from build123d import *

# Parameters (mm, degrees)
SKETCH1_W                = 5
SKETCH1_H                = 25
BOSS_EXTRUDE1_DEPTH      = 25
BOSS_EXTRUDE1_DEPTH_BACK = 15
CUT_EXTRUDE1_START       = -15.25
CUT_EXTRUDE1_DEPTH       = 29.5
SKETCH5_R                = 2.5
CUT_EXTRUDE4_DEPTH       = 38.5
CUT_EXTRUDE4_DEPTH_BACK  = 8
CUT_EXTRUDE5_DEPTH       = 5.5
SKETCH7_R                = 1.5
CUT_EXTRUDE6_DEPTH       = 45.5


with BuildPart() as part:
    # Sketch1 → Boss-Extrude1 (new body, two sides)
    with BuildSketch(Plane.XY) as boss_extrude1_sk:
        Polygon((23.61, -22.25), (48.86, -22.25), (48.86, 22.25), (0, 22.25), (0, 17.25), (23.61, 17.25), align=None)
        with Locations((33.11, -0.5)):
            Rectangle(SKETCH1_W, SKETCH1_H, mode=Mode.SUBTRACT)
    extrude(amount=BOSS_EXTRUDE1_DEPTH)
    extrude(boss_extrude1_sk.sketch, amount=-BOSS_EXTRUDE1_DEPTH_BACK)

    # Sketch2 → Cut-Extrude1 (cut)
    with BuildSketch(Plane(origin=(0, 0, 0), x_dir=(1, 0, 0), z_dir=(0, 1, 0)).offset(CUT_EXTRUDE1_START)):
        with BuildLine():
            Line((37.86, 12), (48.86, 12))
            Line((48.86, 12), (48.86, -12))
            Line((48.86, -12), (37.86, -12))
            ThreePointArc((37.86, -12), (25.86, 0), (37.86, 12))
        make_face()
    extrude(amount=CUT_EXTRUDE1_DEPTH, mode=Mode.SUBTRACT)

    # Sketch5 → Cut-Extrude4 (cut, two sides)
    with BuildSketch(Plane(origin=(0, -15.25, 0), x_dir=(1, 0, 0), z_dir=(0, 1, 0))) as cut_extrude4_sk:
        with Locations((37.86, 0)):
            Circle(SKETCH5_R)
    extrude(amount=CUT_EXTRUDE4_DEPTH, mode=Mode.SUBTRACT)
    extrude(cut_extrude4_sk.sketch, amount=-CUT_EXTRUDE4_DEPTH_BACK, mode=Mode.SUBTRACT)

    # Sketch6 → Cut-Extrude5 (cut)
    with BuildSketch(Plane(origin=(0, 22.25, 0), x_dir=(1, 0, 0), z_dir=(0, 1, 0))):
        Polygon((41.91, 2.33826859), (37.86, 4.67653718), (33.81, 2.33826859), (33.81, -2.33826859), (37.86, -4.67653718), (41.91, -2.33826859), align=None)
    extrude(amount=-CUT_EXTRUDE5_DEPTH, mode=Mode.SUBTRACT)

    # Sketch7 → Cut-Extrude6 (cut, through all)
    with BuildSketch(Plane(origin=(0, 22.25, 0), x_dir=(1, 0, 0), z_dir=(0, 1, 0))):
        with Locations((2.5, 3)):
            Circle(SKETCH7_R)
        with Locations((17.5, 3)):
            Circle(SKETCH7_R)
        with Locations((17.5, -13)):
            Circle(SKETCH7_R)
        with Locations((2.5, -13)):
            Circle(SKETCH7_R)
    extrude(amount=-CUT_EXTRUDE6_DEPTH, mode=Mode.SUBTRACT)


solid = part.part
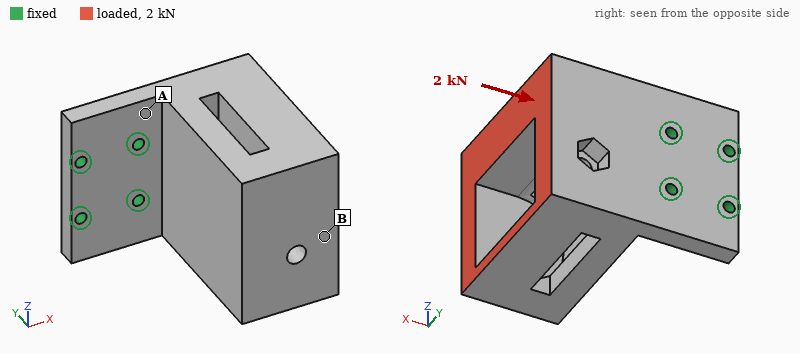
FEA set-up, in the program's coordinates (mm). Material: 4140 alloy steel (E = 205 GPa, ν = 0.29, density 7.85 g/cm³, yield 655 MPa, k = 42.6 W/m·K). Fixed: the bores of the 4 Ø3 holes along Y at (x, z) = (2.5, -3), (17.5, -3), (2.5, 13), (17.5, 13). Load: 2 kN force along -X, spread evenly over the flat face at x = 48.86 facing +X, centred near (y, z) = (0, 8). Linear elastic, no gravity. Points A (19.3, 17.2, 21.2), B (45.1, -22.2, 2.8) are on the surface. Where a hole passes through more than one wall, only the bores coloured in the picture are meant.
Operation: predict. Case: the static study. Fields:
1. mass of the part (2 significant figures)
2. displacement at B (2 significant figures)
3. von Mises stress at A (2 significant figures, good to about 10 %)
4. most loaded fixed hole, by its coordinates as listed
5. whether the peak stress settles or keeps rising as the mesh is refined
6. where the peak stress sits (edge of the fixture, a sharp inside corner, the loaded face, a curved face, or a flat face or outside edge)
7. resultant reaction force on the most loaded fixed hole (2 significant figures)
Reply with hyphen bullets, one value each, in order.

- 250 g
- 0.22 mm
- 170 MPa
- (17.5, 13)
- keeps rising
- edge of the fixture
- 1.2 kN
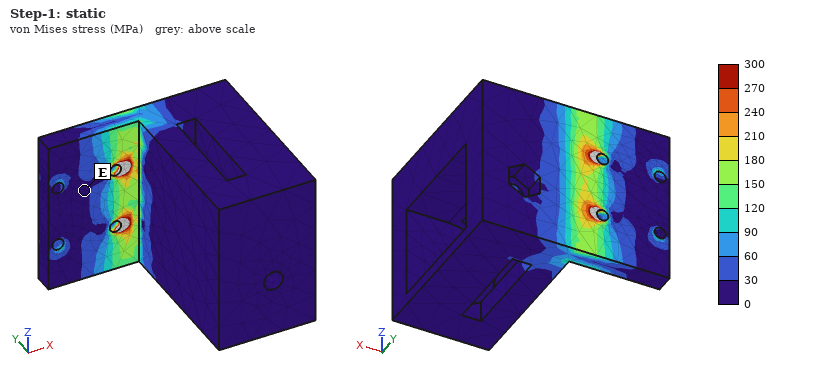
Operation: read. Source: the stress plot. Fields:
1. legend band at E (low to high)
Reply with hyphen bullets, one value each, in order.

- 0 to 30 MPa
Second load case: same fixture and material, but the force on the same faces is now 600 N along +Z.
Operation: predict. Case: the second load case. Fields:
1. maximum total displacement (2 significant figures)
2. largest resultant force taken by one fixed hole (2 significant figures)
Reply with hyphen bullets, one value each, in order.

- 16 µm
- 970 N
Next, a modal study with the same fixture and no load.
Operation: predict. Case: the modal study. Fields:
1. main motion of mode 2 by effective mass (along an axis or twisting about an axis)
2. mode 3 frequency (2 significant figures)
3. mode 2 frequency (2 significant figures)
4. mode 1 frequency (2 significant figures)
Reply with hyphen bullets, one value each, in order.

- along Z
- 5700 Hz
- 2600 Hz
- 1100 Hz
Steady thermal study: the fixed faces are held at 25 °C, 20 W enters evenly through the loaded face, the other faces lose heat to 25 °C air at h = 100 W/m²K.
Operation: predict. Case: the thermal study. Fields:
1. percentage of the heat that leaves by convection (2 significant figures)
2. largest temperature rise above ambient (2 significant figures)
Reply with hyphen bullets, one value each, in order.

- 69 %
- 24 K
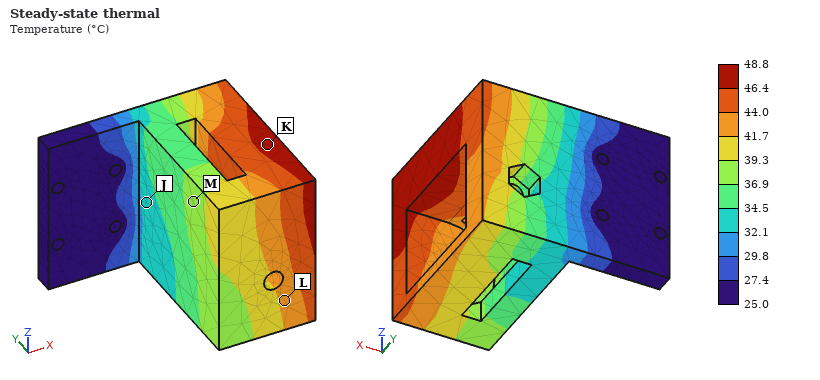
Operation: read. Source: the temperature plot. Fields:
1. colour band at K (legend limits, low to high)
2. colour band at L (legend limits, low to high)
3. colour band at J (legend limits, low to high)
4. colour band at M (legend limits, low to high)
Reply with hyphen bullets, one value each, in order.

- 46.4 to 48.8 °C
- 41.7 to 44.0 °C
- 32.1 to 34.5 °C
- 36.9 to 39.3 °C
